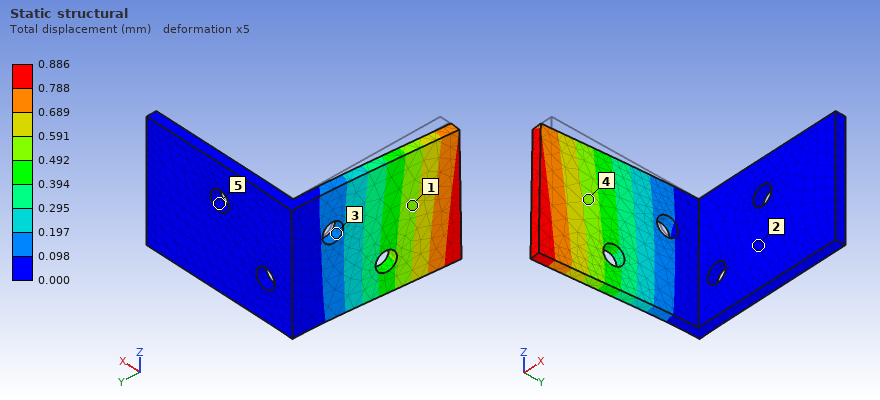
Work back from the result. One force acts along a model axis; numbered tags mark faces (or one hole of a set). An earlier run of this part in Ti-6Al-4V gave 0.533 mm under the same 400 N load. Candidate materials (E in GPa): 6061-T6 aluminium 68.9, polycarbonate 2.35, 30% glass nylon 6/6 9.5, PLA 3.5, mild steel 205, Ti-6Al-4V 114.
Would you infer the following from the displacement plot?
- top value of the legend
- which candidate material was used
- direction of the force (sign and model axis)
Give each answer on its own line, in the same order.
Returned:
0.886 mm
6061-T6 aluminium
-X
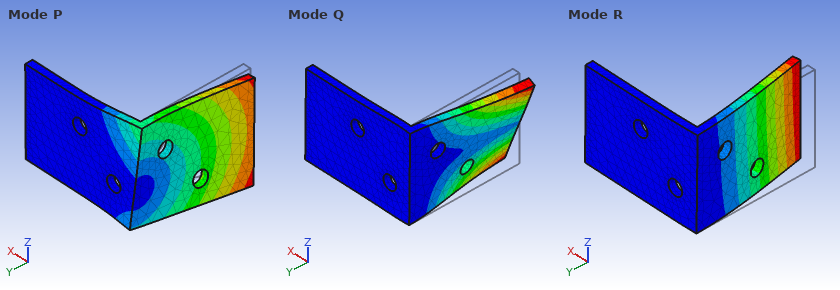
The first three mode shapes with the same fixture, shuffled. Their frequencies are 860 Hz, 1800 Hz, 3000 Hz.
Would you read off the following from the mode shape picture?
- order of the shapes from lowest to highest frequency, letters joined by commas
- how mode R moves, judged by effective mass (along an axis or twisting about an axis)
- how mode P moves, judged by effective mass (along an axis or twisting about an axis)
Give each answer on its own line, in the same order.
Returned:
R, P, Q
along X
along Z
